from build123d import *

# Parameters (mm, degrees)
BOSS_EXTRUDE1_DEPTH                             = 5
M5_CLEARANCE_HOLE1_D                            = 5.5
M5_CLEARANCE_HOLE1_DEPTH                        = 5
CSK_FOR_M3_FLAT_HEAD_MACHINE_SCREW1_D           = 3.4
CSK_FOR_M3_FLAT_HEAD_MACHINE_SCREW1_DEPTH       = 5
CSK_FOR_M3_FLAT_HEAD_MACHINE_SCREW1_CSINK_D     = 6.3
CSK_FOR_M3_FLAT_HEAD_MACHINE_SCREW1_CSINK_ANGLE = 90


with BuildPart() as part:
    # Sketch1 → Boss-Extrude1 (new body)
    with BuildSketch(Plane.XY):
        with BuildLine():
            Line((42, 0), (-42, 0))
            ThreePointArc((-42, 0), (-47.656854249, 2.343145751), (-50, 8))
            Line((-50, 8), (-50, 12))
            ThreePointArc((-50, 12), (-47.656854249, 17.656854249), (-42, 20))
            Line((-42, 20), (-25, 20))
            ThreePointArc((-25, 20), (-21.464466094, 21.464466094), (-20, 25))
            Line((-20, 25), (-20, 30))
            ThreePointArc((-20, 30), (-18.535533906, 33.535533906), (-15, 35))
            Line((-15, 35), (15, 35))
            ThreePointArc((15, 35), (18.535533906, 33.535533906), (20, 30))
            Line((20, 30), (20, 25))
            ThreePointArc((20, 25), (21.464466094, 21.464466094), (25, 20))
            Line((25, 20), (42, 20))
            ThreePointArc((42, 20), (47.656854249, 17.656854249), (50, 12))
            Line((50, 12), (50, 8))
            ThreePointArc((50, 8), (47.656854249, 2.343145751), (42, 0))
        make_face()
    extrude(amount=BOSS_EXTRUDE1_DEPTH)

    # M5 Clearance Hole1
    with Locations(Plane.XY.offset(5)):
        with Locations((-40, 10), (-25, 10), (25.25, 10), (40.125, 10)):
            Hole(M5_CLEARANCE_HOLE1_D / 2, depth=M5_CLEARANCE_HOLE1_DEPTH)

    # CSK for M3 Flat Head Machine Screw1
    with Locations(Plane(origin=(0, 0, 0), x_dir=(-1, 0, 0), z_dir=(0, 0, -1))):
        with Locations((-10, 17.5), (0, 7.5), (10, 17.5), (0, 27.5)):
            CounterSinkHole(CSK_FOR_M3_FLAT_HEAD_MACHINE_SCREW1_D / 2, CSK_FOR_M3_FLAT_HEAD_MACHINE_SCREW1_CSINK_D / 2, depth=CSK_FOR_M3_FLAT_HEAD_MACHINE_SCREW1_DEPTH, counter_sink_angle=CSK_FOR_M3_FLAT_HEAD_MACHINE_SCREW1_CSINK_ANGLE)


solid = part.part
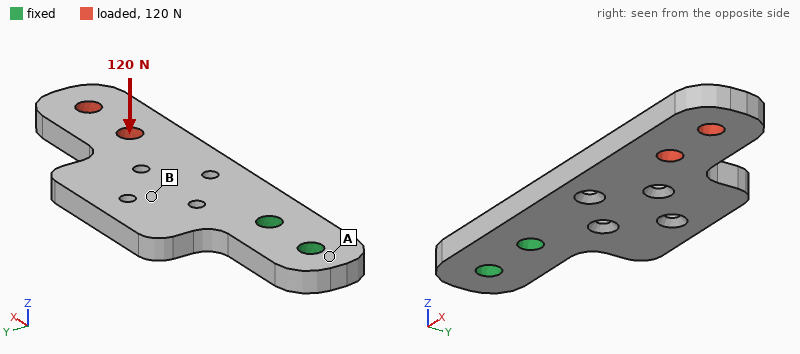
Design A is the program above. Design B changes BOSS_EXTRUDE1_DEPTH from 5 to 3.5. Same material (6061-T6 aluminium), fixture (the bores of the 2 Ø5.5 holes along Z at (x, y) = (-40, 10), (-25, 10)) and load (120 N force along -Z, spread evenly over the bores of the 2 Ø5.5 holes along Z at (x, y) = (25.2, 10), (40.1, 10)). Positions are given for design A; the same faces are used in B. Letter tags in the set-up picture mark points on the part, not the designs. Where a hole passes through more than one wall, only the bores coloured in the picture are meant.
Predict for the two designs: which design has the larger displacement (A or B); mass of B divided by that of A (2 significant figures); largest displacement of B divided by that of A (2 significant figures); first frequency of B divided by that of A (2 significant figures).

B
0.70
2.8
0.71
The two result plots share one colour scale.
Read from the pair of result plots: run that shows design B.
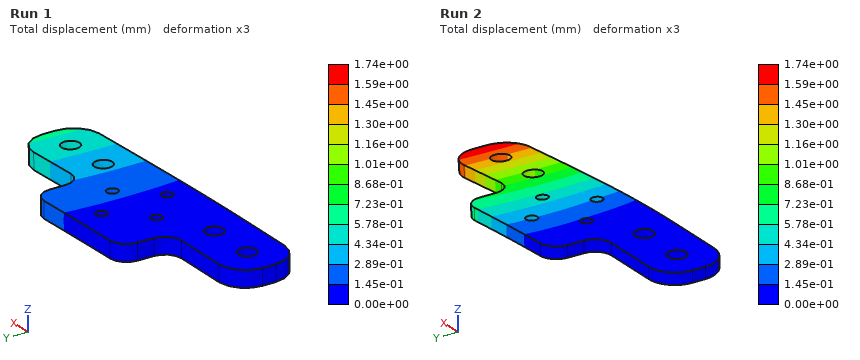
Run 2
